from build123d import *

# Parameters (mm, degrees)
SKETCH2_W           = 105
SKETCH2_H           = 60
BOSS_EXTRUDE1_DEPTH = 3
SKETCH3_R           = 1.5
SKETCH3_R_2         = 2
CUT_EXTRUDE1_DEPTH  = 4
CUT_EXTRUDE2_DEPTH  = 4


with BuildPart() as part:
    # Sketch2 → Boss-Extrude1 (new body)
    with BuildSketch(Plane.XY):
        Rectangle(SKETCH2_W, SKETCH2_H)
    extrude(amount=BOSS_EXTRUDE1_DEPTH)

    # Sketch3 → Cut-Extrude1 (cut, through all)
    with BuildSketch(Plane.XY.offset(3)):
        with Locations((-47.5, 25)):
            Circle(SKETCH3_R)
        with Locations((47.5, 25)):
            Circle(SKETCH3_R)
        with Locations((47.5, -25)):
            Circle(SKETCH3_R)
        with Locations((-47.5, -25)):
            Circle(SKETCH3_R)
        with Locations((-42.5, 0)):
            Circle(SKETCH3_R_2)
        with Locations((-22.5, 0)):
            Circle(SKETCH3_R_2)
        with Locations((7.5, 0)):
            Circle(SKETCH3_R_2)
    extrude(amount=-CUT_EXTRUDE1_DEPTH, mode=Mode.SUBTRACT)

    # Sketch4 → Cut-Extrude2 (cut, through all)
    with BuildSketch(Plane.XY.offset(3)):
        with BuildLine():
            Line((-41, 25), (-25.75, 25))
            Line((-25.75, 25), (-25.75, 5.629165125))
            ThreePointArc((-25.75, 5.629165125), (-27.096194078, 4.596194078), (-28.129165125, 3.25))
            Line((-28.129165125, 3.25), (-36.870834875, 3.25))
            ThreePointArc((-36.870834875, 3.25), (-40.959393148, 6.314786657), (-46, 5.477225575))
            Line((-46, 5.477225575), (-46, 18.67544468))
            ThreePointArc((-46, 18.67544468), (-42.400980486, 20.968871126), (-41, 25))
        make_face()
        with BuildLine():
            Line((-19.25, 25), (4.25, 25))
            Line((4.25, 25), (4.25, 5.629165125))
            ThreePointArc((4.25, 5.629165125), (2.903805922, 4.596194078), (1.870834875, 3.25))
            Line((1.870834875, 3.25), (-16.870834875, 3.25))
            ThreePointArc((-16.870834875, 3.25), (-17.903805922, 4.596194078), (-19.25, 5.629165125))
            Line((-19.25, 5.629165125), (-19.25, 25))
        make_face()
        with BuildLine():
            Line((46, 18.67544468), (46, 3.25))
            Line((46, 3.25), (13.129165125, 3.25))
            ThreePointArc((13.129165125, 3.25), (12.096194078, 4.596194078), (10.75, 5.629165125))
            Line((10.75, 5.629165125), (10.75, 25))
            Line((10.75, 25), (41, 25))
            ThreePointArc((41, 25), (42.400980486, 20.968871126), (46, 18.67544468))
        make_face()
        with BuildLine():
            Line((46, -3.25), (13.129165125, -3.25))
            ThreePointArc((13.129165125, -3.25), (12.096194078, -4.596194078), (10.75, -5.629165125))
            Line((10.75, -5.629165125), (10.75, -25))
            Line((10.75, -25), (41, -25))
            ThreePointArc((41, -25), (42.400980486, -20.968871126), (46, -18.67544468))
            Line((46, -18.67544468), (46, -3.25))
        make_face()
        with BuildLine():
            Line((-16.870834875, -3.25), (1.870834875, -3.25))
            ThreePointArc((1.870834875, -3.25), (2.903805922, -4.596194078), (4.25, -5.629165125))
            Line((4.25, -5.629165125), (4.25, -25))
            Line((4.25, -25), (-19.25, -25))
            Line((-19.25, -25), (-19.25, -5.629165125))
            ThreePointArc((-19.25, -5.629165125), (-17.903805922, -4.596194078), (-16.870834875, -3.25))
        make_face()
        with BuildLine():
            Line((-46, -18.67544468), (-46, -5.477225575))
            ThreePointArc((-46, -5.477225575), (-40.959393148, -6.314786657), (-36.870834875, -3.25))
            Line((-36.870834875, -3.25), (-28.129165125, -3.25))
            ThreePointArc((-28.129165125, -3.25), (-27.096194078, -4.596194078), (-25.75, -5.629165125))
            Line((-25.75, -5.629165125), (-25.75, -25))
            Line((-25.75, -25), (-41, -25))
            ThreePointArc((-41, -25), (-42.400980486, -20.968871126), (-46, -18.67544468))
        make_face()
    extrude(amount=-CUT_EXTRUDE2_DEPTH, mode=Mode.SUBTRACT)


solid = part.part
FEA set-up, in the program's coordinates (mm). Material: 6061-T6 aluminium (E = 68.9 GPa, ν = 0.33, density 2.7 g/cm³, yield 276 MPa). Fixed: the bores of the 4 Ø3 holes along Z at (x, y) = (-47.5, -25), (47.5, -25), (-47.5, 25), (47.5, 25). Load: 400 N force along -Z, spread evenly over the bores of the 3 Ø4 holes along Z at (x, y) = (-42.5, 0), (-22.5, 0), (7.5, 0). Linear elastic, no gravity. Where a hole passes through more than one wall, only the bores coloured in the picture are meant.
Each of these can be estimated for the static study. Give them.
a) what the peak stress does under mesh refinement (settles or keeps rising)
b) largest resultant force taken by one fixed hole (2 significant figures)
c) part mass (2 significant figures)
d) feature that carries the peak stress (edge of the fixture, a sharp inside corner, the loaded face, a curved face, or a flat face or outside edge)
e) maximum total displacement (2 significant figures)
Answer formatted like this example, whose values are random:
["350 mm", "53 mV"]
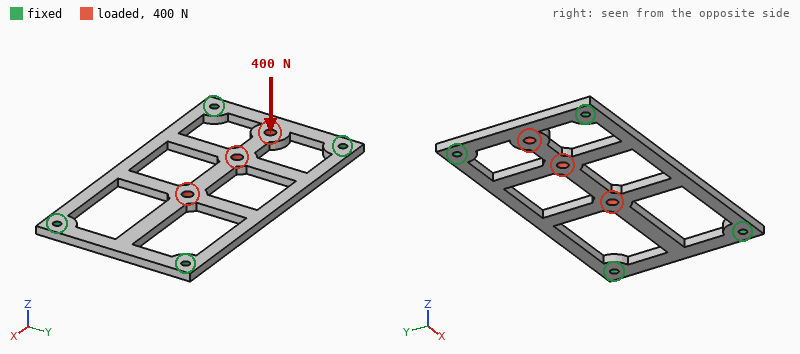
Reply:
["keeps rising", "150 N", "24 g", "edge of the fixture", "0.52 mm"]
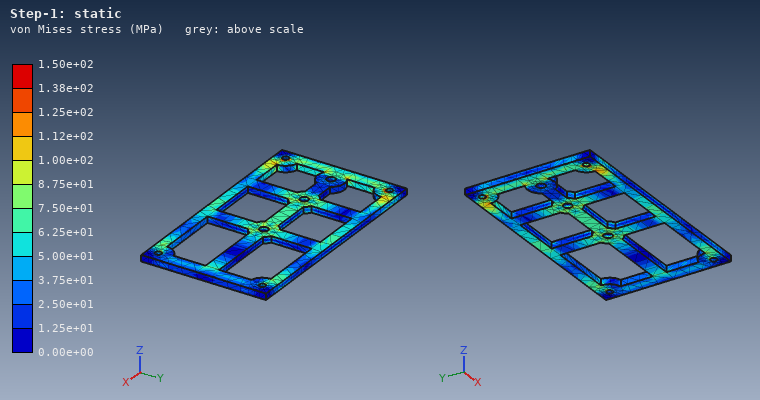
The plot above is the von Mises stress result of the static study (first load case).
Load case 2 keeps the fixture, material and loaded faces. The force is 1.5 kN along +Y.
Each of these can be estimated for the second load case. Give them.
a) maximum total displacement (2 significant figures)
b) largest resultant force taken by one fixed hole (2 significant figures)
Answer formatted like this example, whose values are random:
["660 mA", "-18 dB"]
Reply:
["0.16 mm", "680 N"]
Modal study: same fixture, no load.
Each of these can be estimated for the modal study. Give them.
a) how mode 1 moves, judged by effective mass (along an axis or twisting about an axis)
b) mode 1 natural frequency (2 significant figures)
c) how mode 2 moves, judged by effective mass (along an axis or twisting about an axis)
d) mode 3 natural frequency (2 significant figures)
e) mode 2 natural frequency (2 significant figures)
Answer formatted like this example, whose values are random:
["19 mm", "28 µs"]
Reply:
["along Z", "1300 Hz", "twisting about X", "3300 Hz", "2000 Hz"]
